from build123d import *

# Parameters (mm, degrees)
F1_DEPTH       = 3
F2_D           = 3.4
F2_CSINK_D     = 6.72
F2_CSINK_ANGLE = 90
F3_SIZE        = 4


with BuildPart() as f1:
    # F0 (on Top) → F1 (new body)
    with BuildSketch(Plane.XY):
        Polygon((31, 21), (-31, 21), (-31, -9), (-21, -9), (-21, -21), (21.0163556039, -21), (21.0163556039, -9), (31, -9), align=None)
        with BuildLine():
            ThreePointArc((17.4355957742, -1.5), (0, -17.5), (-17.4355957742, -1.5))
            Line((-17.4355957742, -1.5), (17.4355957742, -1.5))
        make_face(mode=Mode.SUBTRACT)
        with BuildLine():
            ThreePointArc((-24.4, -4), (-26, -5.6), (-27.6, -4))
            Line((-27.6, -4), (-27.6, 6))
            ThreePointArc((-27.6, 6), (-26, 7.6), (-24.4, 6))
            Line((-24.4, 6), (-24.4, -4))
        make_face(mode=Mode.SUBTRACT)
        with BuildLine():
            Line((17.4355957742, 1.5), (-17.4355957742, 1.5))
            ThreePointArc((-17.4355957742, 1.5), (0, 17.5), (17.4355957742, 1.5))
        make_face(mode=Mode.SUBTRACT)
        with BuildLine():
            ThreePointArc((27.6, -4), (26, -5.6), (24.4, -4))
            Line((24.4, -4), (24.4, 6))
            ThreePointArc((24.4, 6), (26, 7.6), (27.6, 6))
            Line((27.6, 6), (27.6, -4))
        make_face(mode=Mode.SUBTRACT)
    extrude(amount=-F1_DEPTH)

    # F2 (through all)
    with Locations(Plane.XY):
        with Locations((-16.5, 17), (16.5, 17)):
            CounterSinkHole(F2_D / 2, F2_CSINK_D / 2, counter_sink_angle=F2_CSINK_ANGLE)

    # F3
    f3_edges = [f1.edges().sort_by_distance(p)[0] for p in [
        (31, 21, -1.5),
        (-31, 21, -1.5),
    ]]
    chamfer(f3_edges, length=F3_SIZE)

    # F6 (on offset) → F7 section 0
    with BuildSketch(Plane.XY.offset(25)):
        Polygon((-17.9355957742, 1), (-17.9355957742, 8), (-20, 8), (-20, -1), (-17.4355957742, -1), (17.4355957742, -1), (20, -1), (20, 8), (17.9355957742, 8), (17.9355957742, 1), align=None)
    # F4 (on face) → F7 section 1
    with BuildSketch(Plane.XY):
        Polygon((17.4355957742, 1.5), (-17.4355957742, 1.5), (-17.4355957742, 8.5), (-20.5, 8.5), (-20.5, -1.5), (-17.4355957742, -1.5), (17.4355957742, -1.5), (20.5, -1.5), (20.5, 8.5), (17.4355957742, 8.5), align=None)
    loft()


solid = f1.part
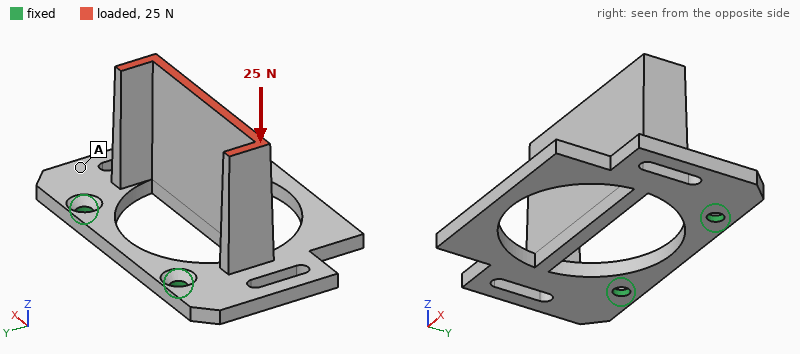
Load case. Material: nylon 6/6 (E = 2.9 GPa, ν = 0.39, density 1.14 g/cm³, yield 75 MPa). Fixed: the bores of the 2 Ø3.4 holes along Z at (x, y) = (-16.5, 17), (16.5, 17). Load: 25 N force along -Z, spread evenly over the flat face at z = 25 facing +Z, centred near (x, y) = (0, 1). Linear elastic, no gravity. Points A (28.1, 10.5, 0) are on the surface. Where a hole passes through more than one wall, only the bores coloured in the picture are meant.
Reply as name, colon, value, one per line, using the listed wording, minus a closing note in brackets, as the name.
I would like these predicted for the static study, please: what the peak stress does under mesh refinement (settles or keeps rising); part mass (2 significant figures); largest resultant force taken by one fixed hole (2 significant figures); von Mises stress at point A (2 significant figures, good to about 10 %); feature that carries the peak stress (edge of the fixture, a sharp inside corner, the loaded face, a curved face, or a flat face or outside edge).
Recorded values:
what the peak stress does under mesh refinement: keeps rising
part mass: 8.6 g
largest resultant force taken by one fixed hole: 13 N
von Mises stress at point A: 2.7 MPa
feature that carries the peak stress: edge of the fixture
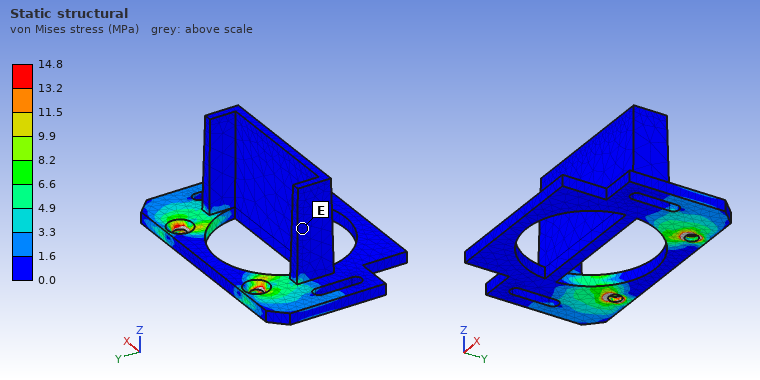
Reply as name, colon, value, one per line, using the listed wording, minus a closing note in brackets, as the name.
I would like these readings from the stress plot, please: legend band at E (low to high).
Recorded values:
legend band at E: 0.0 to 1.6 MPa
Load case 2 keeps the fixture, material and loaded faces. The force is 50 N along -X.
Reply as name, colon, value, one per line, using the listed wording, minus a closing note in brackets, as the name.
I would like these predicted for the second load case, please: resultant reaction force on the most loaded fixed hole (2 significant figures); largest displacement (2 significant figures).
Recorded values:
resultant reaction force on the most loaded fixed hole: 43 N
largest displacement: 0.92 mm
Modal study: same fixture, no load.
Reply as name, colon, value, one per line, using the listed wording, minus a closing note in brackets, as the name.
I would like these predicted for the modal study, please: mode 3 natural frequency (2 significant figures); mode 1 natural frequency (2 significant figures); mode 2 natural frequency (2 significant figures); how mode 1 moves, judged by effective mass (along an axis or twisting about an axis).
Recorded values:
mode 3 natural frequency: 1200 Hz
mode 1 natural frequency: 320 Hz
mode 2 natural frequency: 690 Hz
how mode 1 moves, judged by effective mass: along Z
